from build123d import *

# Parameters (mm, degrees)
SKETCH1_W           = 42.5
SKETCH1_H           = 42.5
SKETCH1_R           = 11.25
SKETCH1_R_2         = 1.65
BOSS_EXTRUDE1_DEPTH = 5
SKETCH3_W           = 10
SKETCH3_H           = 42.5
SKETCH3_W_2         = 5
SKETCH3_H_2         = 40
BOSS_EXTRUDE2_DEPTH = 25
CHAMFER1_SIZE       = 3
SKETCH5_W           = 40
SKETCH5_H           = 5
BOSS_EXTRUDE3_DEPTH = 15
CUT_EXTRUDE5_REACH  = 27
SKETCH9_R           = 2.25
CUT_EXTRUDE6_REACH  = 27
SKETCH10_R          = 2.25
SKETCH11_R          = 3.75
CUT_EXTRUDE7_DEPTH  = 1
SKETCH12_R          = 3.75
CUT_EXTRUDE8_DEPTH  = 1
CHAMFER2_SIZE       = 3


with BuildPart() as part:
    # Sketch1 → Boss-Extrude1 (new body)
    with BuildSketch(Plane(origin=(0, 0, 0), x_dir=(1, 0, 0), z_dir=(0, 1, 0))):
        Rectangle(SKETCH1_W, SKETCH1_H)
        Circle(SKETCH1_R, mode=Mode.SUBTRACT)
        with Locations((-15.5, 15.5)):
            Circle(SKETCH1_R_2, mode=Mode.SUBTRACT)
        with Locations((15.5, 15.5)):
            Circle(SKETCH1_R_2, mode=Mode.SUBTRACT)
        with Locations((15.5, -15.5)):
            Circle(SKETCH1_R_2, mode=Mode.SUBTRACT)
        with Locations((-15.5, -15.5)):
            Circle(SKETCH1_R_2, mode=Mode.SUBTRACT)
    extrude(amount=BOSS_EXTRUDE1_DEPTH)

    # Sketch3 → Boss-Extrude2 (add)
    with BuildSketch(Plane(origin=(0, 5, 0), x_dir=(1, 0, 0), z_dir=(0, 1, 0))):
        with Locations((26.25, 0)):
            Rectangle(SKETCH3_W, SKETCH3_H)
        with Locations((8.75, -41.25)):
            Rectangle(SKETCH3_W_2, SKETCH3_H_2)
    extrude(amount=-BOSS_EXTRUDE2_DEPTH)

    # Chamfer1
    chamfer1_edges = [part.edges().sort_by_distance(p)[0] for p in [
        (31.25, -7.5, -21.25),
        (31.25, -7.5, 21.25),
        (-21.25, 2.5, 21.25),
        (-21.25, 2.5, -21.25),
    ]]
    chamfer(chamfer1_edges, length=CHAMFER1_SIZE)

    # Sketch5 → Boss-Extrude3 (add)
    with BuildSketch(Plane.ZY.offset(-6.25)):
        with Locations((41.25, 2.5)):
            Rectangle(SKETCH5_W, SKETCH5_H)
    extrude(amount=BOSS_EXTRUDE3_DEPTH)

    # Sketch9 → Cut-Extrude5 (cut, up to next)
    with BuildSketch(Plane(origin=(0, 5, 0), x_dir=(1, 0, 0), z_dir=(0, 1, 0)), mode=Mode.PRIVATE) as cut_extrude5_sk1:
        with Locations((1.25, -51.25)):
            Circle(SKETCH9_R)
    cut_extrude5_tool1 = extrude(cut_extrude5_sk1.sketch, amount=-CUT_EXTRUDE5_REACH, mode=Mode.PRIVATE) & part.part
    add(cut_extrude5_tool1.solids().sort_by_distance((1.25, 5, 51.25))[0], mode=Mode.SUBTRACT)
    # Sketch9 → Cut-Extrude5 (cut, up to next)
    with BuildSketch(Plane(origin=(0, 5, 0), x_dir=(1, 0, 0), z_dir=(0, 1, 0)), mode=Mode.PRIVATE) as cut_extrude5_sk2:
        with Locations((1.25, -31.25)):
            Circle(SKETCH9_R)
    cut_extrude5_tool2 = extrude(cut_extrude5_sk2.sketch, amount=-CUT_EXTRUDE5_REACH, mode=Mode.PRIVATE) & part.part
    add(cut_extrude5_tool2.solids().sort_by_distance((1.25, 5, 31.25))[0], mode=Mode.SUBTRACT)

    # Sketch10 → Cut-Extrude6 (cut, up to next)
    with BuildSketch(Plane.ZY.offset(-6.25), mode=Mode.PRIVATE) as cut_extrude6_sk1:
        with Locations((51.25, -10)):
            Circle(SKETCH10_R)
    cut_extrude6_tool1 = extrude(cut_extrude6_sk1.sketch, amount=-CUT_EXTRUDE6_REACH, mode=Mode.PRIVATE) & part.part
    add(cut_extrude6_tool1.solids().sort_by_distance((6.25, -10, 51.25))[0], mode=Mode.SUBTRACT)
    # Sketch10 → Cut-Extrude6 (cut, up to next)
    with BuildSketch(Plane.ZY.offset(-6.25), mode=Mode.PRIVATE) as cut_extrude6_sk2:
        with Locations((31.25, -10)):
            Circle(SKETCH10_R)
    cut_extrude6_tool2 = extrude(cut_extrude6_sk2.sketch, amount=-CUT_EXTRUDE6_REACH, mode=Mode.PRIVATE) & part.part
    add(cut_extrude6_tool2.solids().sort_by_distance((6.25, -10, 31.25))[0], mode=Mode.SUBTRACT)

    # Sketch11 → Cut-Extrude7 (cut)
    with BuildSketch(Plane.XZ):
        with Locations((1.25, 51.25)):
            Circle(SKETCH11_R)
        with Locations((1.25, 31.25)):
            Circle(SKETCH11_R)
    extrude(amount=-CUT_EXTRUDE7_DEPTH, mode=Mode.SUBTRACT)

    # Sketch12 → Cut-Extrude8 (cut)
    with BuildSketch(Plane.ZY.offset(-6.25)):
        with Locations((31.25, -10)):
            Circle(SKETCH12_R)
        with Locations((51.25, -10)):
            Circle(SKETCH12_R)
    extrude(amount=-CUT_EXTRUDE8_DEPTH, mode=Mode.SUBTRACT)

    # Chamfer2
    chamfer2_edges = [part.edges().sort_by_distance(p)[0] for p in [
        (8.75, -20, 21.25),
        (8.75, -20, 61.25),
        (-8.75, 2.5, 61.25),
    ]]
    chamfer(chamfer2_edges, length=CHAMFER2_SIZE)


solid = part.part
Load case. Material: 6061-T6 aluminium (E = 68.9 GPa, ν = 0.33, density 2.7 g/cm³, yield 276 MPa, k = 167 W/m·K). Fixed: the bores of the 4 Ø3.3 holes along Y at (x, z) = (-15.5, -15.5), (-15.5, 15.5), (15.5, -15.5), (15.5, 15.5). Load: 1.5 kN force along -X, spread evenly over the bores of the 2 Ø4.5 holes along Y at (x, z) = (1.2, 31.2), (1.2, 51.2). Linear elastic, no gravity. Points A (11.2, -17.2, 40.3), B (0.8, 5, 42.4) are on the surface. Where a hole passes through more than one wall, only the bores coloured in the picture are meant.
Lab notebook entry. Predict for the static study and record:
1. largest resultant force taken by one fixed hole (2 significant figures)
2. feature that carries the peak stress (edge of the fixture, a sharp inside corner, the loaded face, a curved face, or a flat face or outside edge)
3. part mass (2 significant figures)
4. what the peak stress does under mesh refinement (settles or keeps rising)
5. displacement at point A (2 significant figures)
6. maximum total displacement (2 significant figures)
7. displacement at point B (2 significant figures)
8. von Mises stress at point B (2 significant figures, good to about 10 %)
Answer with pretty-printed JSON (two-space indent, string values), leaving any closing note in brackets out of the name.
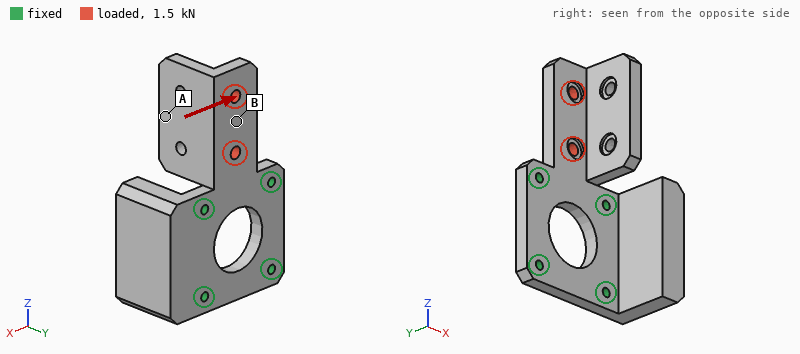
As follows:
{
  "largest resultant force taken by one fixed hole": "1.5 kN",
  "feature that carries the peak stress": "a sharp inside corner",
  "part mass": "67 g",
  "what the peak stress does under mesh refinement": "keeps rising",
  "displacement at point A": "0.037 mm",
  "maximum total displacement": "0.11 mm",
  "displacement at point B": "0.056 mm",
  "von Mises stress at point B": "26 MPa"
}
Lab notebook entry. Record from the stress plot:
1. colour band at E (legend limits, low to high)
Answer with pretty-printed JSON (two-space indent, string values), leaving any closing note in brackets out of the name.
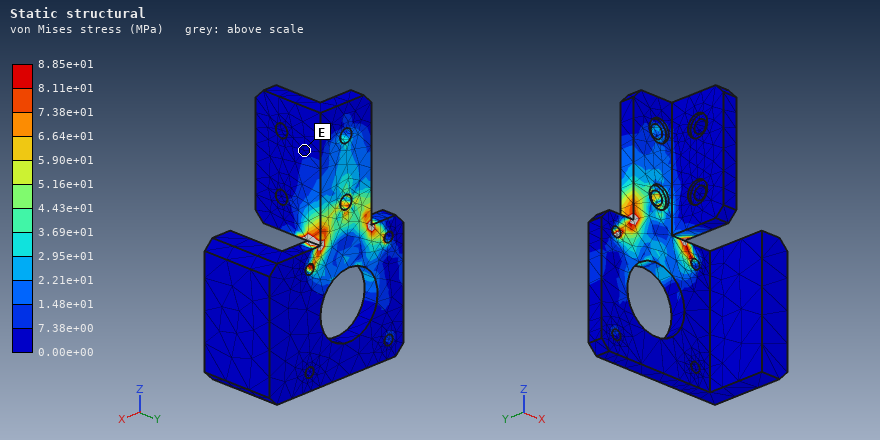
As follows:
{
  "colour band at E": "0.00e+00 to 7.38e+00 MPa"
}
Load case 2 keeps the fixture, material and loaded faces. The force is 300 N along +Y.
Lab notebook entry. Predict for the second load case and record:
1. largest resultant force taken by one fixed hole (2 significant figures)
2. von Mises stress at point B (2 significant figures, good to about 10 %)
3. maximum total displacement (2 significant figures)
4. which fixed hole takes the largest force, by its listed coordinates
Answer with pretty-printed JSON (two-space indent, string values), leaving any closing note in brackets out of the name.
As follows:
{
  "largest resultant force taken by one fixed hole": "220 N",
  "von Mises stress at point B": "11 MPa",
  "maximum total displacement": "0.29 mm",
  "which fixed hole takes the largest force, by its listed coordinates": "(15.5, 15.5)"
}
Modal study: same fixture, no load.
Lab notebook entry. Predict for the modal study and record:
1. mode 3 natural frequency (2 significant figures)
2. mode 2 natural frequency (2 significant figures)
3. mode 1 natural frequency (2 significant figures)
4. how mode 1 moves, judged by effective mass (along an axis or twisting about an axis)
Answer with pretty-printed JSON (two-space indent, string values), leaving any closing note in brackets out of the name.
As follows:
{
  "mode 3 natural frequency": "3600 Hz",
  "mode 2 natural frequency": "3300 Hz",
  "mode 1 natural frequency": "1300 Hz",
  "how mode 1 moves, judged by effective mass": "along Y"
}
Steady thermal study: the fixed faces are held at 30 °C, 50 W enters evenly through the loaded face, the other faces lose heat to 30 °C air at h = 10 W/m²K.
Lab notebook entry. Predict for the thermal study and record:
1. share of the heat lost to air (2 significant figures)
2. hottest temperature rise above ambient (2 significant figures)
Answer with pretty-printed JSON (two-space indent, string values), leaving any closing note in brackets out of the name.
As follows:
{
  "share of the heat lost to air": "4.9 %",
  "hottest temperature rise above ambient": "78 K"
}
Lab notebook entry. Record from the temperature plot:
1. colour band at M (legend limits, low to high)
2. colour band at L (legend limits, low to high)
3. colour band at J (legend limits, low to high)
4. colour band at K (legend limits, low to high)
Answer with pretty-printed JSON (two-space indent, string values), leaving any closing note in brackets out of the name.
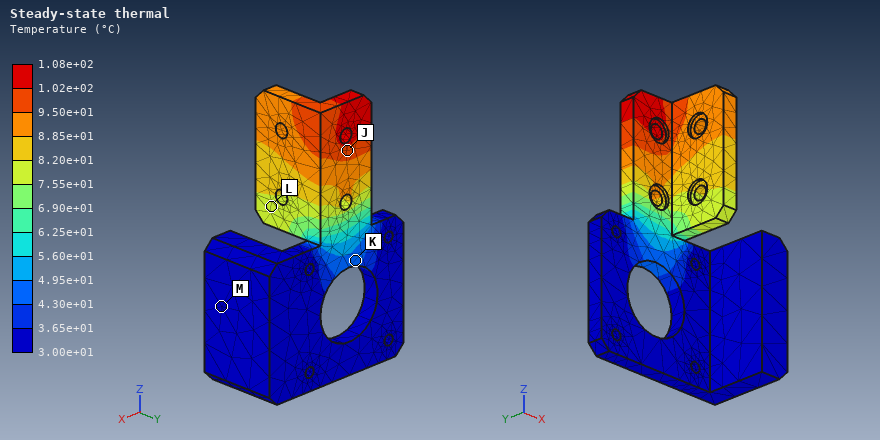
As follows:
{
  "colour band at M": "3.00e+01 to 3.65e+01 °C",
  "colour band at L": "7.55e+01 to 8.20e+01 °C",
  "colour band at J": "9.50e+01 to 1.02e+02 °C",
  "colour band at K": "4.30e+01 to 4.95e+01 °C"
}
